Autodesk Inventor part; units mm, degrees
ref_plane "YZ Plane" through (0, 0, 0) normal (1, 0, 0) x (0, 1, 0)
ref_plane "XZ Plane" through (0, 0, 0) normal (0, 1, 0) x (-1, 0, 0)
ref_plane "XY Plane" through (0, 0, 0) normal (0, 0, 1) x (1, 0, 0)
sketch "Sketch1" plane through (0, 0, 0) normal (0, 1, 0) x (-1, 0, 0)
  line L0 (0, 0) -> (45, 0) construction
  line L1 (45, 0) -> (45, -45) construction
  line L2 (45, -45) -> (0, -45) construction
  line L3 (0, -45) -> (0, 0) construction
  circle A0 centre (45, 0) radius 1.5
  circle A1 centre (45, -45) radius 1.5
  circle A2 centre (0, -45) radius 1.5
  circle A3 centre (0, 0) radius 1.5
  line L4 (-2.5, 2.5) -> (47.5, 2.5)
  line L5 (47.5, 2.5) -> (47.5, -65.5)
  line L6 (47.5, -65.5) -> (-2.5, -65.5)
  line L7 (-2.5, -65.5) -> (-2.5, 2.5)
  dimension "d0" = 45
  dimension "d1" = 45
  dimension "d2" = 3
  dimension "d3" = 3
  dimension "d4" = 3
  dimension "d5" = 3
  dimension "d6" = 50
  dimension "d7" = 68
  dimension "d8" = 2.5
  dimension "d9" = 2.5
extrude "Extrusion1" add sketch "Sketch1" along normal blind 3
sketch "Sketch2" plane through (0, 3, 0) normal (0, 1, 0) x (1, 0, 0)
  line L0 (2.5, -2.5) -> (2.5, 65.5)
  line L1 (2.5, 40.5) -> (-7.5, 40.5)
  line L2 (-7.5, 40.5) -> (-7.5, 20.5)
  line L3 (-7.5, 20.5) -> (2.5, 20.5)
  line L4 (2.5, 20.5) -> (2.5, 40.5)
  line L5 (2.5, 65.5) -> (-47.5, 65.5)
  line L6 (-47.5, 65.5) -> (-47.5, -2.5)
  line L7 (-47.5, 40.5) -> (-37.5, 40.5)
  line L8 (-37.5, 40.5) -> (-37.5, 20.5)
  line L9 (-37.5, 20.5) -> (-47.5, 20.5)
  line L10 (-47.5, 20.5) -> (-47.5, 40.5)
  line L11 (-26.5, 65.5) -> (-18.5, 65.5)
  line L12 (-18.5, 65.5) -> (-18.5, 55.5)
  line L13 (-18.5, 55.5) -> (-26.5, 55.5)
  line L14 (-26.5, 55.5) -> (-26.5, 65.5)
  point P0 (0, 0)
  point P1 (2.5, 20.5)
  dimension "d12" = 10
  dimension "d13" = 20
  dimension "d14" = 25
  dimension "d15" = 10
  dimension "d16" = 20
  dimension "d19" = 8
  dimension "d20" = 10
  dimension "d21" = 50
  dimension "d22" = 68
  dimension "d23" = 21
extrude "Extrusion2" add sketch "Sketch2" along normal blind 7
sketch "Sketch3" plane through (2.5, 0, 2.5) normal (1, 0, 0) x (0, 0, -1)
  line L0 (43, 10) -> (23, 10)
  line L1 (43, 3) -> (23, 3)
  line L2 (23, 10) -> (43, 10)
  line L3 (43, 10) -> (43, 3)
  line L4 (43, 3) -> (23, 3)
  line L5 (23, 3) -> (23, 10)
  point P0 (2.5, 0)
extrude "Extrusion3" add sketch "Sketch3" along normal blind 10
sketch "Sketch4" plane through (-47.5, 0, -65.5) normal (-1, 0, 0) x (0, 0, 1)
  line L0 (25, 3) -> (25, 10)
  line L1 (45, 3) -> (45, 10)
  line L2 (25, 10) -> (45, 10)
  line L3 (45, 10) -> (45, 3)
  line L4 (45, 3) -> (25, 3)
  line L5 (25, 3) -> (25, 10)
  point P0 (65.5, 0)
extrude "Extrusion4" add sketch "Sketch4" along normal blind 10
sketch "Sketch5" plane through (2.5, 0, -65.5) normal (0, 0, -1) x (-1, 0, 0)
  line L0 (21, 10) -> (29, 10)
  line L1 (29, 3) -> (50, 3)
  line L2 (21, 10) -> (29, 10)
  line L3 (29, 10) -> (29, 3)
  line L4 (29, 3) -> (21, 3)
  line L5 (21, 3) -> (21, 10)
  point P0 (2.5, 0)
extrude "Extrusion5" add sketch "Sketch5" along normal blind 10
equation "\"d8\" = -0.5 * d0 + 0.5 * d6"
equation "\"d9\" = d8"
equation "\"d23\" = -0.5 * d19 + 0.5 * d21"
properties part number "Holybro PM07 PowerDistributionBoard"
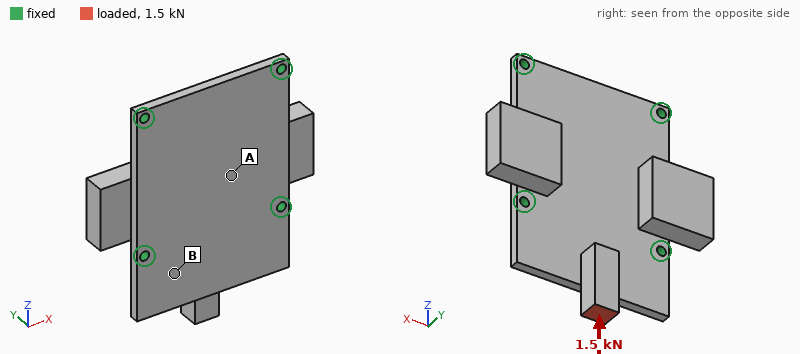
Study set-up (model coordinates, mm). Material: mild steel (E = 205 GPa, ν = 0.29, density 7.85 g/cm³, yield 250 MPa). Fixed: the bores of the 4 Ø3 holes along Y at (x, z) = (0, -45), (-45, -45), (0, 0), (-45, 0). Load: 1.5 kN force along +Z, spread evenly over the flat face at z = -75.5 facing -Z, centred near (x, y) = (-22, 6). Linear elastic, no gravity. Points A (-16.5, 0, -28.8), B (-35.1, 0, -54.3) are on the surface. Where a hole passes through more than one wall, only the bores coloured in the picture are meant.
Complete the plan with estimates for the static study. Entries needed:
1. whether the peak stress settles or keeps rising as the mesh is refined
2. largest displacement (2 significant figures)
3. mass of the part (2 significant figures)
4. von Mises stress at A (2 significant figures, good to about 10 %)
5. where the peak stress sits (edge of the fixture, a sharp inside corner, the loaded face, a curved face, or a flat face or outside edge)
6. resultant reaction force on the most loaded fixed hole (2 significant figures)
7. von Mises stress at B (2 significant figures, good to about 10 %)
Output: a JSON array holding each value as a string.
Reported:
["keeps rising", "0.18 mm", "130 g", "16 MPa", "edge of the fixture", "530 N", "84 MPa"]
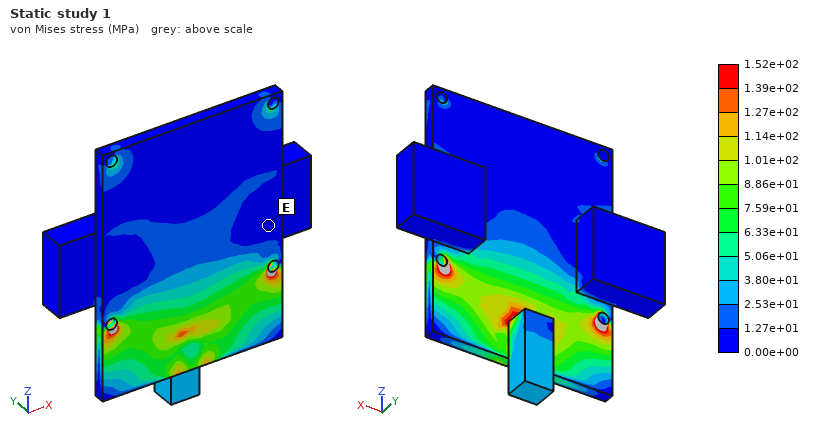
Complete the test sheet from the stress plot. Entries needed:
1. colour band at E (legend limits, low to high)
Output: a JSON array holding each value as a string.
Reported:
["0.00e+00 to 1.27e+01 MPa"]
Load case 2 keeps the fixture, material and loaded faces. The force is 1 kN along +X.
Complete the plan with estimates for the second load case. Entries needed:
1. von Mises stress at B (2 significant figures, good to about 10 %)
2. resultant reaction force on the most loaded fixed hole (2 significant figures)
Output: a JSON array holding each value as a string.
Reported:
["27 MPa", "820 N"]
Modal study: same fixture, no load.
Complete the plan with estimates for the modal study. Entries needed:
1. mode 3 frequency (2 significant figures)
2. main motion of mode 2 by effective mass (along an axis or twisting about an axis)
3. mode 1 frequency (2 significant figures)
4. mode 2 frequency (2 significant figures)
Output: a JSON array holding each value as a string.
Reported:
["5100 Hz", "along Y", "2500 Hz", "4600 Hz"]
